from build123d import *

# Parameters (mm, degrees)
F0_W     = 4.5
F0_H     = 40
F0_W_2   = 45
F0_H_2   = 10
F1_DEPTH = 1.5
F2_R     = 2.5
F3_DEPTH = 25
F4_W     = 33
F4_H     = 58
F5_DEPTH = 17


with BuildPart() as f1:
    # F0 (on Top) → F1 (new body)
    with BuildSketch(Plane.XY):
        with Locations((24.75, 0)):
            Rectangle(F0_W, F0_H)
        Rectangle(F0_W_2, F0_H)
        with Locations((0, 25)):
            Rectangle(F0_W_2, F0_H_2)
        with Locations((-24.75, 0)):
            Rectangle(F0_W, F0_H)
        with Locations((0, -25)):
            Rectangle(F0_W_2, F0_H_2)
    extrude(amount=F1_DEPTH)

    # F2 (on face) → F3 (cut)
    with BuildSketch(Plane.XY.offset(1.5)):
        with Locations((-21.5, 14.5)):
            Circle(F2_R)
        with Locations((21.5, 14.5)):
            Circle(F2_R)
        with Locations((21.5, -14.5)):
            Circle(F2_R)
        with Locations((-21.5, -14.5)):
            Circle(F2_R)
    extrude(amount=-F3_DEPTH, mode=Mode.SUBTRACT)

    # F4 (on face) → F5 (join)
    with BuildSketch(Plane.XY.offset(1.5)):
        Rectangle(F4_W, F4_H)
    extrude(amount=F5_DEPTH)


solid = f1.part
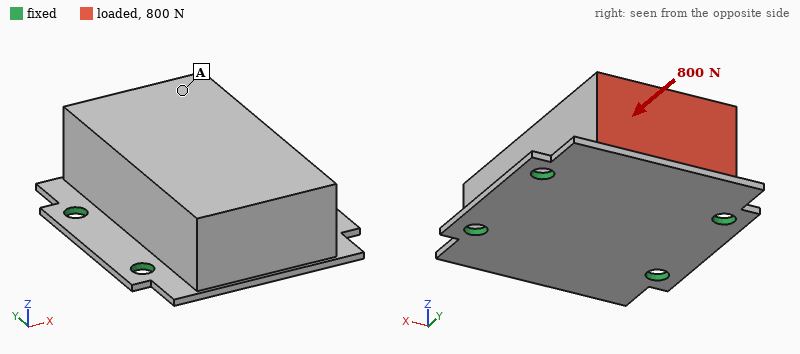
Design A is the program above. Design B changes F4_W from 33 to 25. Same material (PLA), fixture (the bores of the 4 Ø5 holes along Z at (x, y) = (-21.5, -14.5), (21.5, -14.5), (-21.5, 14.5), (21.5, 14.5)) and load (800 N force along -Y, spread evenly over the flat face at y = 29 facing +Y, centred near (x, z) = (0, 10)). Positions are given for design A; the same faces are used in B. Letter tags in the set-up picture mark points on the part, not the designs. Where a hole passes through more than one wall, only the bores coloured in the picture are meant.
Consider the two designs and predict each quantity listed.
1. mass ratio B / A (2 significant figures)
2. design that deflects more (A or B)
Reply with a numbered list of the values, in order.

1. 0.79
2. B
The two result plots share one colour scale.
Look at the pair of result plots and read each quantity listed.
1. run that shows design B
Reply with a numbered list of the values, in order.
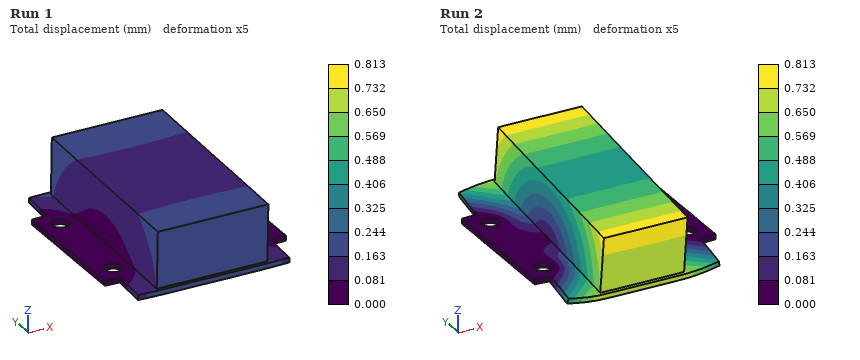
1. Run 2
